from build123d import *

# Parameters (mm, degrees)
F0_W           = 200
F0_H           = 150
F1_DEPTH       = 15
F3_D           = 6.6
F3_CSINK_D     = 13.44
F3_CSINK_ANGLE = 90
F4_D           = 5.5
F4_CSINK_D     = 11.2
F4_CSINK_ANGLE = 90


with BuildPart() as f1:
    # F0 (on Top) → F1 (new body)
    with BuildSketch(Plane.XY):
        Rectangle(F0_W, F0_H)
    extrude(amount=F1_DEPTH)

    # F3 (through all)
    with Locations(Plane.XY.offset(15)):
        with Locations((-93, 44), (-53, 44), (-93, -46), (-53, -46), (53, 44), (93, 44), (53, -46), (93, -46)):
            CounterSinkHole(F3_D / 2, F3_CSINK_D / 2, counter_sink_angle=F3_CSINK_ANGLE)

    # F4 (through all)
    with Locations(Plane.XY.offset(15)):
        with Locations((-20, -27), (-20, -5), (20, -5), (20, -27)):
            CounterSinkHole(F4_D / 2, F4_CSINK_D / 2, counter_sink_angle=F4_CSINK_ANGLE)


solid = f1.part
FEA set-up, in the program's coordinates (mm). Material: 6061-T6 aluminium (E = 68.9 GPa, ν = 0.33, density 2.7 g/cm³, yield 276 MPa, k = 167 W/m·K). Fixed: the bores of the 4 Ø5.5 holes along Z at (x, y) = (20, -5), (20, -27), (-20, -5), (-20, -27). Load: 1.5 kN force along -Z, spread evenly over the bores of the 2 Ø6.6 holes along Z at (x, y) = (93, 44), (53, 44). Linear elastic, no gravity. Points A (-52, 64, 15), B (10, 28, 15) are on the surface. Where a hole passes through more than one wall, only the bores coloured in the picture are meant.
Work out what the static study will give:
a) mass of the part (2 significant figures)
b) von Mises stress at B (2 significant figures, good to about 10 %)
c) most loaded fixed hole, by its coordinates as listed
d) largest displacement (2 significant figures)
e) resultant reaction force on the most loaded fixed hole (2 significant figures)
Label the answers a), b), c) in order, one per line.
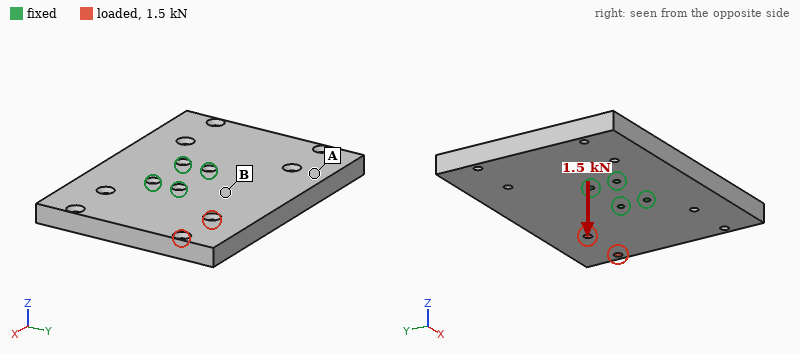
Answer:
a) 1.2 kg
b) 14 MPa
c) (20, -5)
d) 0.21 mm
e) 3.2 kN
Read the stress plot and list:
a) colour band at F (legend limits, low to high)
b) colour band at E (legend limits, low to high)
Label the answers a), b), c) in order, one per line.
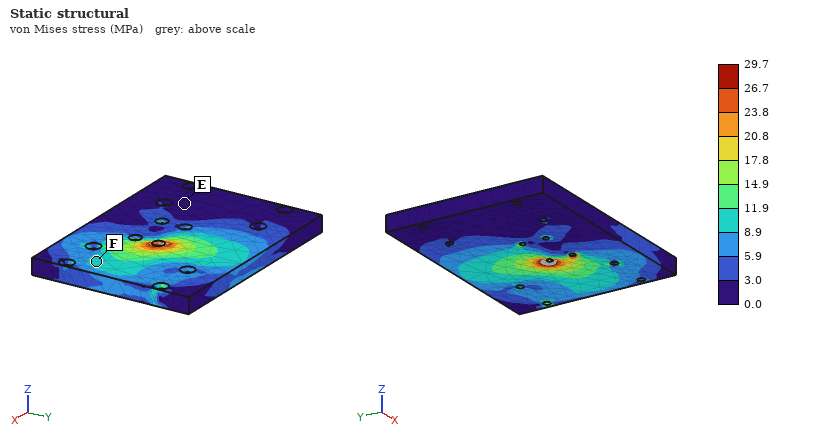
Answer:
a) 8.9 to 11.9 MPa
b) 0.0 to 3.0 MPa
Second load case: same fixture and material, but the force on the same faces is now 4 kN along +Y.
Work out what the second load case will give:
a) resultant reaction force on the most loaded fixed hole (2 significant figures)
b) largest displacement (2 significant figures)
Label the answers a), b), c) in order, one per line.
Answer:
a) 4.2 kN
b) 30 µm
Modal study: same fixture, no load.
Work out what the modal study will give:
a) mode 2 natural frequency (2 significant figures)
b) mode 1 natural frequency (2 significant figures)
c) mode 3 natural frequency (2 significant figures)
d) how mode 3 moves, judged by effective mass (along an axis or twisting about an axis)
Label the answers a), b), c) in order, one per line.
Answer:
a) 1200 Hz
b) 1200 Hz
c) 1700 Hz
d) along Z
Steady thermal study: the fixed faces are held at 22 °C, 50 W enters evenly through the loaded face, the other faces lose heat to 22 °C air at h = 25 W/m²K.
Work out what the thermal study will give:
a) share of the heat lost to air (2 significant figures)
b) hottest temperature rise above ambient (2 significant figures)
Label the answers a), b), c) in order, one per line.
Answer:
a) 15 %
b) 19 K
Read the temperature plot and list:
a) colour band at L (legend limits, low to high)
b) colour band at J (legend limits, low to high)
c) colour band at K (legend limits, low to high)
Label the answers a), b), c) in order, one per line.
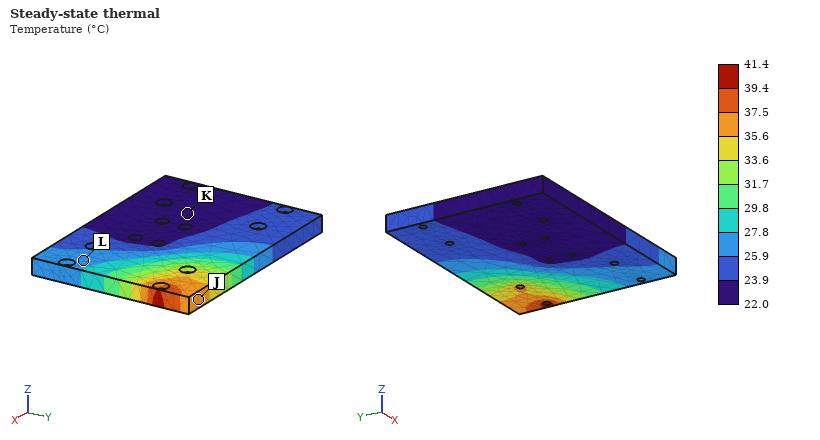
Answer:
a) 25.9 to 27.8 °C
b) 35.6 to 37.5 °C
c) 22.0 to 23.9 °C
